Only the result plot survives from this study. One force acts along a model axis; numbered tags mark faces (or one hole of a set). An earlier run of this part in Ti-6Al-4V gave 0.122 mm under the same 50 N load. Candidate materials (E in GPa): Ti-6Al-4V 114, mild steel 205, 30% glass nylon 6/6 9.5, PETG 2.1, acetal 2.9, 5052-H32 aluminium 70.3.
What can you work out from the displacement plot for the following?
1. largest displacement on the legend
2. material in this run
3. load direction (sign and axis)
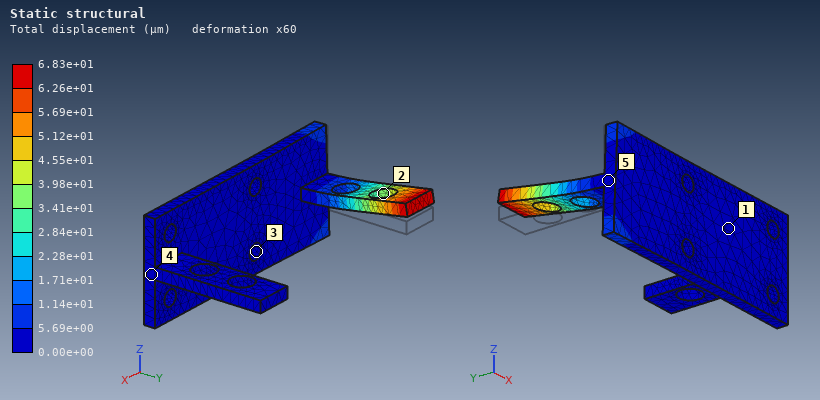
6.83e+01 µm
mild steel
+Z
